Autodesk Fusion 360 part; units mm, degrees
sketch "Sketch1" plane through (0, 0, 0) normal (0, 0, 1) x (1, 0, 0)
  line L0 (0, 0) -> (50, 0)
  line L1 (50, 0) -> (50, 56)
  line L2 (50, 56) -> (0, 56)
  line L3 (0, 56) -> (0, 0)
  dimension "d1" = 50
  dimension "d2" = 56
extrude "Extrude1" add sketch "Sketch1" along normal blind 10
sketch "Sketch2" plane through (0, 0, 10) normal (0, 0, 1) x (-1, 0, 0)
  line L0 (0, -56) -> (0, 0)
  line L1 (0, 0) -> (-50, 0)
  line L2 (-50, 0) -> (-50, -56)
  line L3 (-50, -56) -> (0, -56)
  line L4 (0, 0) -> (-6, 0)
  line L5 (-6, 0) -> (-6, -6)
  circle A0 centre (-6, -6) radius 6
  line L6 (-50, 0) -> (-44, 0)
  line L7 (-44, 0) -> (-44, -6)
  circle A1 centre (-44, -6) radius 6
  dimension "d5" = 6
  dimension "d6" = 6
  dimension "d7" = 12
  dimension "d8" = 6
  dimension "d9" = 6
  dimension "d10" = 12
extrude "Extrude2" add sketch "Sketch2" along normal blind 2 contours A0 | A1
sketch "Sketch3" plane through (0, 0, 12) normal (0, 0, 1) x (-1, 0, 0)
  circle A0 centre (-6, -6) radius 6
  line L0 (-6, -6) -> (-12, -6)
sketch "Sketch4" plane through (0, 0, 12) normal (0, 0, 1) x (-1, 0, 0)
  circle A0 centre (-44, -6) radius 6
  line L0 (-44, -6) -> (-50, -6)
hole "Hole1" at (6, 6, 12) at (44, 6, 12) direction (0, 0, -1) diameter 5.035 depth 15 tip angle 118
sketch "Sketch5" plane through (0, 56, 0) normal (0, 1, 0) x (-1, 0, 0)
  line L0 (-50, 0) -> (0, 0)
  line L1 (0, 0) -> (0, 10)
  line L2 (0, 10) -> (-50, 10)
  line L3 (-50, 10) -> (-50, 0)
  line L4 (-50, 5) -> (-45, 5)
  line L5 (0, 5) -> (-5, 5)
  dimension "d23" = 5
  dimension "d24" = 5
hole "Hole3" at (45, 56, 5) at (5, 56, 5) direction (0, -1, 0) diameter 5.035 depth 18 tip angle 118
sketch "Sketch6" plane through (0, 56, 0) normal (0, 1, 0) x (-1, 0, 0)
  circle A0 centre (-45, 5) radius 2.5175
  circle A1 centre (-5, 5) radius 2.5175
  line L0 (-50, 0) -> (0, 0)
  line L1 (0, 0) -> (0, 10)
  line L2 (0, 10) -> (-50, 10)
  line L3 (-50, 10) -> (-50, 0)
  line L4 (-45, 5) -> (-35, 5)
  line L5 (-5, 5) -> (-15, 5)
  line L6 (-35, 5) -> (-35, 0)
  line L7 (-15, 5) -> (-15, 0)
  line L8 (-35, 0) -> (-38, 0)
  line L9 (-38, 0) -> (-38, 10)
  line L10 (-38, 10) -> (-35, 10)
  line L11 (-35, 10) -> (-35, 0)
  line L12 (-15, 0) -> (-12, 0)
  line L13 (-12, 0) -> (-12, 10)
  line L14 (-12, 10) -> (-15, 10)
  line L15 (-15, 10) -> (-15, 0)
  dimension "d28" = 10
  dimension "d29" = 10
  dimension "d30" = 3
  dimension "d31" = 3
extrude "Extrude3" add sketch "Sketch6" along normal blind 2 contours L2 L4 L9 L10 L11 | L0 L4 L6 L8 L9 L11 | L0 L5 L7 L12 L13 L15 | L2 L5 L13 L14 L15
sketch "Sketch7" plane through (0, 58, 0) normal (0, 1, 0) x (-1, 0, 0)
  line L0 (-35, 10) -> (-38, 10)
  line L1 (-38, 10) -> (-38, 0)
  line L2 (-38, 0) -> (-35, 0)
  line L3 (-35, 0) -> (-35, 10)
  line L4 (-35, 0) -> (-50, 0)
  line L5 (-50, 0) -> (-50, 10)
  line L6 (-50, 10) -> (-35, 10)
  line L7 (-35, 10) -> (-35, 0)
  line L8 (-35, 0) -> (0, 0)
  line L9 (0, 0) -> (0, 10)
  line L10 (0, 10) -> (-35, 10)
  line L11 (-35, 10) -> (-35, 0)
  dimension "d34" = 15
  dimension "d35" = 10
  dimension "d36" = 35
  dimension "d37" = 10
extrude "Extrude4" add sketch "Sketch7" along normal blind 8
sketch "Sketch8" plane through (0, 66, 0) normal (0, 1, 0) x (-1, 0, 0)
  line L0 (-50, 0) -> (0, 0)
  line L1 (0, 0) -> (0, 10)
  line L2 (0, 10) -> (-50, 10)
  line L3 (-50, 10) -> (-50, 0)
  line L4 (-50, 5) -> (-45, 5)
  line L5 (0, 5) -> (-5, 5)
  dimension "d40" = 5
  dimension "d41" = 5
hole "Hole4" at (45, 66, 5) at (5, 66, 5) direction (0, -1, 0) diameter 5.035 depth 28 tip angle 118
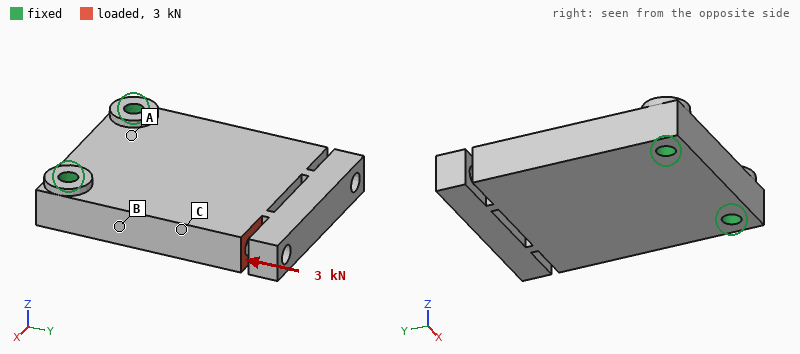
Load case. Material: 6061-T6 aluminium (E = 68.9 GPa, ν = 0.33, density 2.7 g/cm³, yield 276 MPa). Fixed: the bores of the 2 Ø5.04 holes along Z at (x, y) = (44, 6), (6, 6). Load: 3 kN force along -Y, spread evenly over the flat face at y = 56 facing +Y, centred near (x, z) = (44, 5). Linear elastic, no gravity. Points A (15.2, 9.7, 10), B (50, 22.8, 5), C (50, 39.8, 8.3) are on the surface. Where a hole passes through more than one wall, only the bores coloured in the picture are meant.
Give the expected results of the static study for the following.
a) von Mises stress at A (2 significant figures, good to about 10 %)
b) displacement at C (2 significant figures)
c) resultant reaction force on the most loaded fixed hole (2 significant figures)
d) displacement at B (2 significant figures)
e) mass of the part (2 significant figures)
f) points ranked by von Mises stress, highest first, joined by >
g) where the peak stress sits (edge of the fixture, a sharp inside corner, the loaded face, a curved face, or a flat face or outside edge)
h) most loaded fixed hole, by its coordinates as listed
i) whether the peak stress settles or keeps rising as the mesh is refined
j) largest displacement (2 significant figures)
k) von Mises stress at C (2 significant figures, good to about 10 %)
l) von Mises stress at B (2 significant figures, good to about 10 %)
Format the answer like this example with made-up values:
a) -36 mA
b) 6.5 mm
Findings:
a) 4.2 MPa
b) 13 µm
c) 3.0 kN
d) 5.7 µm
e) 84 g
f) C > B > A
g) edge of the fixture
h) (44, 6)
i) keeps rising
j) 23 µm
k) 28 MPa
l) 22 MPa
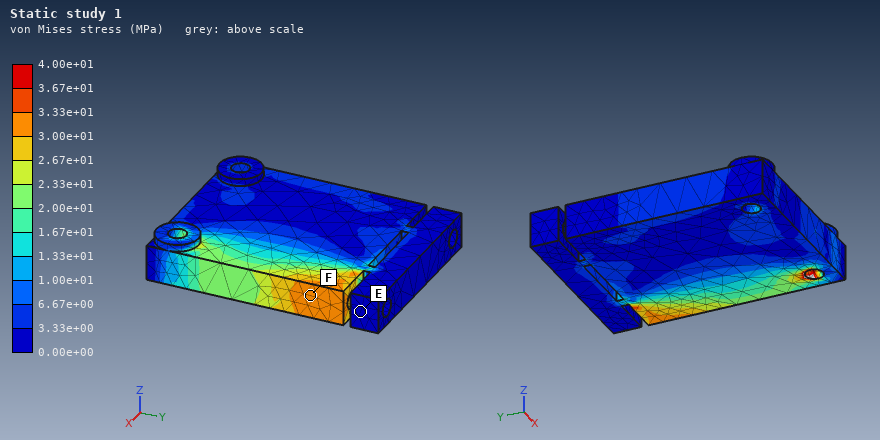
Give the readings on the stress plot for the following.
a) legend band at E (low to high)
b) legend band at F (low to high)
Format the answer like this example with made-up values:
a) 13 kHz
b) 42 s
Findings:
a) 0.00e+00 to 3.33e+00 MPa
b) 3.00e+01 to 3.33e+01 MPa
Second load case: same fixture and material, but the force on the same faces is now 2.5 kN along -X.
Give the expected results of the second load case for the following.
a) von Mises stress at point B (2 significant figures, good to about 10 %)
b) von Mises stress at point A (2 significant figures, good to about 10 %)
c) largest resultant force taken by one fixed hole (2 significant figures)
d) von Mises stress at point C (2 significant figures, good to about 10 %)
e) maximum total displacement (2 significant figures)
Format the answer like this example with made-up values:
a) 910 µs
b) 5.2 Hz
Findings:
a) 21 MPa
b) 11 MPa
c) 3.4 kN
d) 23 MPa
e) 47 µm
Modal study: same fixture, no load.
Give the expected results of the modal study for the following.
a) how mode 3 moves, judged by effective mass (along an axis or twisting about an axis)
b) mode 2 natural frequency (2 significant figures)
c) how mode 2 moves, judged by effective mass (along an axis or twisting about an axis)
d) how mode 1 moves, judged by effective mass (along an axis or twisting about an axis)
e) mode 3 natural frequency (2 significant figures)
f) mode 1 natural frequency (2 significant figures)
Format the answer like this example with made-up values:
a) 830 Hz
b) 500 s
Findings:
a) along X
b) 6100 Hz
c) twisting about Y
d) along Z
e) 8300 Hz
f) 2200 Hz
